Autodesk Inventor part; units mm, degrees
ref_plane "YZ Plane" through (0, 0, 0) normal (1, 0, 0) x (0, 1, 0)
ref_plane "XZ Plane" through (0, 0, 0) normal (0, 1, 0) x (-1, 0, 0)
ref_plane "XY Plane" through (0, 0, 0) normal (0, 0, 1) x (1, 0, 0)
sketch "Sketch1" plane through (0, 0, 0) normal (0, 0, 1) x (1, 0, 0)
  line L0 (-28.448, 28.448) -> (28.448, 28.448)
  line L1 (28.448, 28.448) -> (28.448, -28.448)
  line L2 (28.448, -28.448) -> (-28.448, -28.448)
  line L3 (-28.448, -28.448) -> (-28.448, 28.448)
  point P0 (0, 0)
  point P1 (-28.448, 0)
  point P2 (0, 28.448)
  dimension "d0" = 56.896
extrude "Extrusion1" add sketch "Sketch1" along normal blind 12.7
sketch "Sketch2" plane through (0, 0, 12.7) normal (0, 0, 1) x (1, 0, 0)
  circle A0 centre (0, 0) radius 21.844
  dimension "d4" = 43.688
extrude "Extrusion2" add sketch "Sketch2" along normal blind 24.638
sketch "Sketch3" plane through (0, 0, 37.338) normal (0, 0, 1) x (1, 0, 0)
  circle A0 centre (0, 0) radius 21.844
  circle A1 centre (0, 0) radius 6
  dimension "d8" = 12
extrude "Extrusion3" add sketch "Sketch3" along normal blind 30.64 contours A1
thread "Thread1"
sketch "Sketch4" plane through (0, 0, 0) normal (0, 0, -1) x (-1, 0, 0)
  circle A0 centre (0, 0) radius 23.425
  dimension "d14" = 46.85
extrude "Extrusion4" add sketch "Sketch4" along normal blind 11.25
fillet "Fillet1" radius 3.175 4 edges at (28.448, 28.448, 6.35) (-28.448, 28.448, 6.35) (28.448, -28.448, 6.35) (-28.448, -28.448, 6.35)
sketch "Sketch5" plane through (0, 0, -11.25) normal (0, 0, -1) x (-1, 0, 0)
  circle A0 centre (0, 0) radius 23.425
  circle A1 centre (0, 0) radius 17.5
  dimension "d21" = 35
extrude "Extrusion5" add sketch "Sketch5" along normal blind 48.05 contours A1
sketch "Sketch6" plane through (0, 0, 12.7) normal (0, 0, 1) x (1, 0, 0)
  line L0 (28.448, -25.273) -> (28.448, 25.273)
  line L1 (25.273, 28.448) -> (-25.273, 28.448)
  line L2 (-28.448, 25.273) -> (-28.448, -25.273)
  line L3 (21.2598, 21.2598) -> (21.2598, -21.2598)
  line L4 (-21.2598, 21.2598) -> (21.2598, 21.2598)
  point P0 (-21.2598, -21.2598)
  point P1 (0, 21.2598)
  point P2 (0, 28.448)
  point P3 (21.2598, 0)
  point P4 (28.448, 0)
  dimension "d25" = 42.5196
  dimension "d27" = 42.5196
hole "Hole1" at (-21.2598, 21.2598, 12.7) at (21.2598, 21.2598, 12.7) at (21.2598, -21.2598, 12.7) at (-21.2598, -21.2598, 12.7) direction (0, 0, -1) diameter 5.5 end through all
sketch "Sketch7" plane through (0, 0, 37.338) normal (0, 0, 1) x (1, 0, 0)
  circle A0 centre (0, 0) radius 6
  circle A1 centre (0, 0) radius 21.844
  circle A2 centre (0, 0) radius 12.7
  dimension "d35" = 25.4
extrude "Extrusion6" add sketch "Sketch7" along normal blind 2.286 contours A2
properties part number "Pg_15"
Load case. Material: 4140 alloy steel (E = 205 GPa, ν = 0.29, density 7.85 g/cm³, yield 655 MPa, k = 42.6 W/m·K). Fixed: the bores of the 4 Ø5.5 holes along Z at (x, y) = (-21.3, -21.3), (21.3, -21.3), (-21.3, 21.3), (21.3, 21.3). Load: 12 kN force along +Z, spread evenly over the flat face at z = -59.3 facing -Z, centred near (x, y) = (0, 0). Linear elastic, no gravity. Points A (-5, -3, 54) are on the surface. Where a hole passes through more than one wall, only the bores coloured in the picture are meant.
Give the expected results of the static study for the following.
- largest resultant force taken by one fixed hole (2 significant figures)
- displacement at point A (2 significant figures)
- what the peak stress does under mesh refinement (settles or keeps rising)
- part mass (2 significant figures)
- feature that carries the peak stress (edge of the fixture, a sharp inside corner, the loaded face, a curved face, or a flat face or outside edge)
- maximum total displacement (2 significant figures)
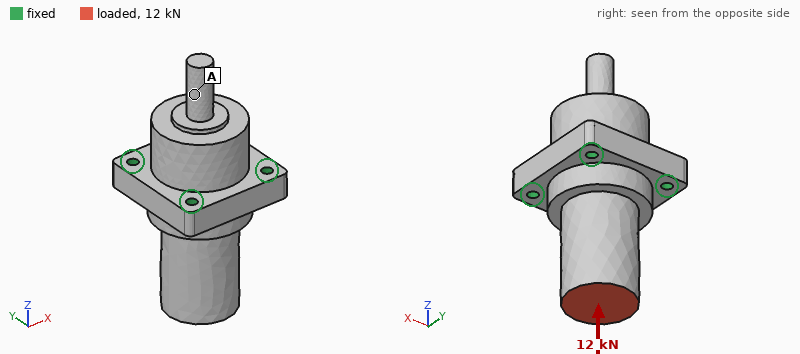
3.0 kN
1.9 µm
keeps rising
1.2 kg
edge of the fixture
5.6 µm
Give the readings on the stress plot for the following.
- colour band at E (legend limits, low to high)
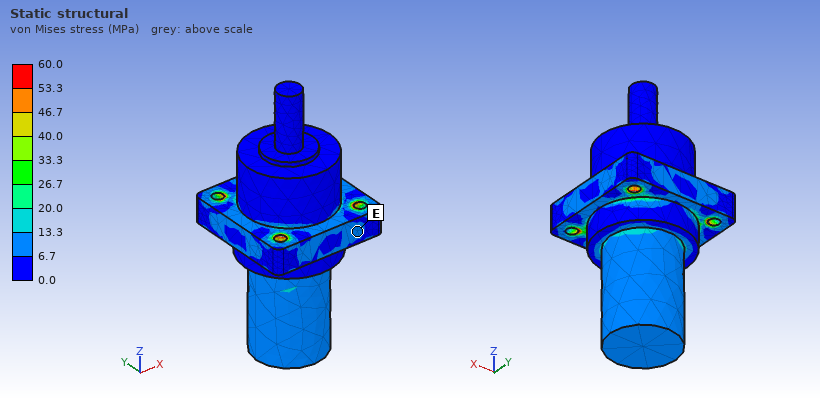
6.7 to 13.3 MPa
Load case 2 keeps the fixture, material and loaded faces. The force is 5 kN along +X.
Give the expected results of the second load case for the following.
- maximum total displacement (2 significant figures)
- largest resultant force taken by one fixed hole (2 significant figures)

34 µm
4.2 kN
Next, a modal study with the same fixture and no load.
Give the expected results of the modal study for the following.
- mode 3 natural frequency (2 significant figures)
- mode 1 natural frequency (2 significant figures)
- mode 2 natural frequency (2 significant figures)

7900 Hz
5300 Hz
5300 Hz
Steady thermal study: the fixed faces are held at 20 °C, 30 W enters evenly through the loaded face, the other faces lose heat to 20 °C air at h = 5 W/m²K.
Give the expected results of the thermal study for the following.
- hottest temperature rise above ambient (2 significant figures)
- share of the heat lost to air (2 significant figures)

48 K
4.0 %
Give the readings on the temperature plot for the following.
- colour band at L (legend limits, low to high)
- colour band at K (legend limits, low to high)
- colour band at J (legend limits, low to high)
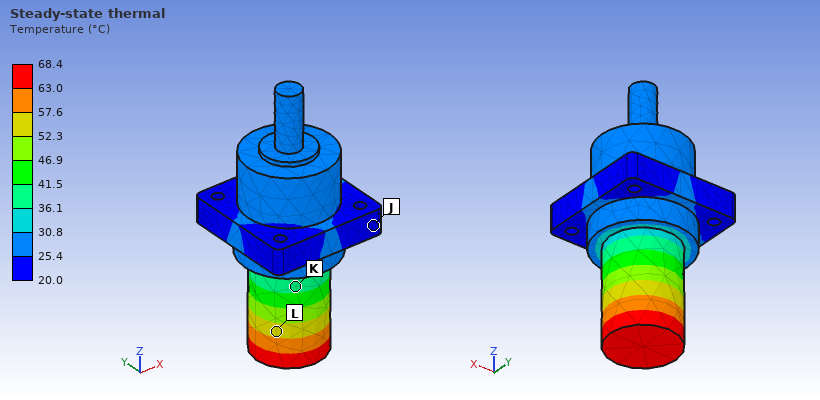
52.3 to 57.6 °C
36.1 to 41.5 °C
20.0 to 25.4 °C
